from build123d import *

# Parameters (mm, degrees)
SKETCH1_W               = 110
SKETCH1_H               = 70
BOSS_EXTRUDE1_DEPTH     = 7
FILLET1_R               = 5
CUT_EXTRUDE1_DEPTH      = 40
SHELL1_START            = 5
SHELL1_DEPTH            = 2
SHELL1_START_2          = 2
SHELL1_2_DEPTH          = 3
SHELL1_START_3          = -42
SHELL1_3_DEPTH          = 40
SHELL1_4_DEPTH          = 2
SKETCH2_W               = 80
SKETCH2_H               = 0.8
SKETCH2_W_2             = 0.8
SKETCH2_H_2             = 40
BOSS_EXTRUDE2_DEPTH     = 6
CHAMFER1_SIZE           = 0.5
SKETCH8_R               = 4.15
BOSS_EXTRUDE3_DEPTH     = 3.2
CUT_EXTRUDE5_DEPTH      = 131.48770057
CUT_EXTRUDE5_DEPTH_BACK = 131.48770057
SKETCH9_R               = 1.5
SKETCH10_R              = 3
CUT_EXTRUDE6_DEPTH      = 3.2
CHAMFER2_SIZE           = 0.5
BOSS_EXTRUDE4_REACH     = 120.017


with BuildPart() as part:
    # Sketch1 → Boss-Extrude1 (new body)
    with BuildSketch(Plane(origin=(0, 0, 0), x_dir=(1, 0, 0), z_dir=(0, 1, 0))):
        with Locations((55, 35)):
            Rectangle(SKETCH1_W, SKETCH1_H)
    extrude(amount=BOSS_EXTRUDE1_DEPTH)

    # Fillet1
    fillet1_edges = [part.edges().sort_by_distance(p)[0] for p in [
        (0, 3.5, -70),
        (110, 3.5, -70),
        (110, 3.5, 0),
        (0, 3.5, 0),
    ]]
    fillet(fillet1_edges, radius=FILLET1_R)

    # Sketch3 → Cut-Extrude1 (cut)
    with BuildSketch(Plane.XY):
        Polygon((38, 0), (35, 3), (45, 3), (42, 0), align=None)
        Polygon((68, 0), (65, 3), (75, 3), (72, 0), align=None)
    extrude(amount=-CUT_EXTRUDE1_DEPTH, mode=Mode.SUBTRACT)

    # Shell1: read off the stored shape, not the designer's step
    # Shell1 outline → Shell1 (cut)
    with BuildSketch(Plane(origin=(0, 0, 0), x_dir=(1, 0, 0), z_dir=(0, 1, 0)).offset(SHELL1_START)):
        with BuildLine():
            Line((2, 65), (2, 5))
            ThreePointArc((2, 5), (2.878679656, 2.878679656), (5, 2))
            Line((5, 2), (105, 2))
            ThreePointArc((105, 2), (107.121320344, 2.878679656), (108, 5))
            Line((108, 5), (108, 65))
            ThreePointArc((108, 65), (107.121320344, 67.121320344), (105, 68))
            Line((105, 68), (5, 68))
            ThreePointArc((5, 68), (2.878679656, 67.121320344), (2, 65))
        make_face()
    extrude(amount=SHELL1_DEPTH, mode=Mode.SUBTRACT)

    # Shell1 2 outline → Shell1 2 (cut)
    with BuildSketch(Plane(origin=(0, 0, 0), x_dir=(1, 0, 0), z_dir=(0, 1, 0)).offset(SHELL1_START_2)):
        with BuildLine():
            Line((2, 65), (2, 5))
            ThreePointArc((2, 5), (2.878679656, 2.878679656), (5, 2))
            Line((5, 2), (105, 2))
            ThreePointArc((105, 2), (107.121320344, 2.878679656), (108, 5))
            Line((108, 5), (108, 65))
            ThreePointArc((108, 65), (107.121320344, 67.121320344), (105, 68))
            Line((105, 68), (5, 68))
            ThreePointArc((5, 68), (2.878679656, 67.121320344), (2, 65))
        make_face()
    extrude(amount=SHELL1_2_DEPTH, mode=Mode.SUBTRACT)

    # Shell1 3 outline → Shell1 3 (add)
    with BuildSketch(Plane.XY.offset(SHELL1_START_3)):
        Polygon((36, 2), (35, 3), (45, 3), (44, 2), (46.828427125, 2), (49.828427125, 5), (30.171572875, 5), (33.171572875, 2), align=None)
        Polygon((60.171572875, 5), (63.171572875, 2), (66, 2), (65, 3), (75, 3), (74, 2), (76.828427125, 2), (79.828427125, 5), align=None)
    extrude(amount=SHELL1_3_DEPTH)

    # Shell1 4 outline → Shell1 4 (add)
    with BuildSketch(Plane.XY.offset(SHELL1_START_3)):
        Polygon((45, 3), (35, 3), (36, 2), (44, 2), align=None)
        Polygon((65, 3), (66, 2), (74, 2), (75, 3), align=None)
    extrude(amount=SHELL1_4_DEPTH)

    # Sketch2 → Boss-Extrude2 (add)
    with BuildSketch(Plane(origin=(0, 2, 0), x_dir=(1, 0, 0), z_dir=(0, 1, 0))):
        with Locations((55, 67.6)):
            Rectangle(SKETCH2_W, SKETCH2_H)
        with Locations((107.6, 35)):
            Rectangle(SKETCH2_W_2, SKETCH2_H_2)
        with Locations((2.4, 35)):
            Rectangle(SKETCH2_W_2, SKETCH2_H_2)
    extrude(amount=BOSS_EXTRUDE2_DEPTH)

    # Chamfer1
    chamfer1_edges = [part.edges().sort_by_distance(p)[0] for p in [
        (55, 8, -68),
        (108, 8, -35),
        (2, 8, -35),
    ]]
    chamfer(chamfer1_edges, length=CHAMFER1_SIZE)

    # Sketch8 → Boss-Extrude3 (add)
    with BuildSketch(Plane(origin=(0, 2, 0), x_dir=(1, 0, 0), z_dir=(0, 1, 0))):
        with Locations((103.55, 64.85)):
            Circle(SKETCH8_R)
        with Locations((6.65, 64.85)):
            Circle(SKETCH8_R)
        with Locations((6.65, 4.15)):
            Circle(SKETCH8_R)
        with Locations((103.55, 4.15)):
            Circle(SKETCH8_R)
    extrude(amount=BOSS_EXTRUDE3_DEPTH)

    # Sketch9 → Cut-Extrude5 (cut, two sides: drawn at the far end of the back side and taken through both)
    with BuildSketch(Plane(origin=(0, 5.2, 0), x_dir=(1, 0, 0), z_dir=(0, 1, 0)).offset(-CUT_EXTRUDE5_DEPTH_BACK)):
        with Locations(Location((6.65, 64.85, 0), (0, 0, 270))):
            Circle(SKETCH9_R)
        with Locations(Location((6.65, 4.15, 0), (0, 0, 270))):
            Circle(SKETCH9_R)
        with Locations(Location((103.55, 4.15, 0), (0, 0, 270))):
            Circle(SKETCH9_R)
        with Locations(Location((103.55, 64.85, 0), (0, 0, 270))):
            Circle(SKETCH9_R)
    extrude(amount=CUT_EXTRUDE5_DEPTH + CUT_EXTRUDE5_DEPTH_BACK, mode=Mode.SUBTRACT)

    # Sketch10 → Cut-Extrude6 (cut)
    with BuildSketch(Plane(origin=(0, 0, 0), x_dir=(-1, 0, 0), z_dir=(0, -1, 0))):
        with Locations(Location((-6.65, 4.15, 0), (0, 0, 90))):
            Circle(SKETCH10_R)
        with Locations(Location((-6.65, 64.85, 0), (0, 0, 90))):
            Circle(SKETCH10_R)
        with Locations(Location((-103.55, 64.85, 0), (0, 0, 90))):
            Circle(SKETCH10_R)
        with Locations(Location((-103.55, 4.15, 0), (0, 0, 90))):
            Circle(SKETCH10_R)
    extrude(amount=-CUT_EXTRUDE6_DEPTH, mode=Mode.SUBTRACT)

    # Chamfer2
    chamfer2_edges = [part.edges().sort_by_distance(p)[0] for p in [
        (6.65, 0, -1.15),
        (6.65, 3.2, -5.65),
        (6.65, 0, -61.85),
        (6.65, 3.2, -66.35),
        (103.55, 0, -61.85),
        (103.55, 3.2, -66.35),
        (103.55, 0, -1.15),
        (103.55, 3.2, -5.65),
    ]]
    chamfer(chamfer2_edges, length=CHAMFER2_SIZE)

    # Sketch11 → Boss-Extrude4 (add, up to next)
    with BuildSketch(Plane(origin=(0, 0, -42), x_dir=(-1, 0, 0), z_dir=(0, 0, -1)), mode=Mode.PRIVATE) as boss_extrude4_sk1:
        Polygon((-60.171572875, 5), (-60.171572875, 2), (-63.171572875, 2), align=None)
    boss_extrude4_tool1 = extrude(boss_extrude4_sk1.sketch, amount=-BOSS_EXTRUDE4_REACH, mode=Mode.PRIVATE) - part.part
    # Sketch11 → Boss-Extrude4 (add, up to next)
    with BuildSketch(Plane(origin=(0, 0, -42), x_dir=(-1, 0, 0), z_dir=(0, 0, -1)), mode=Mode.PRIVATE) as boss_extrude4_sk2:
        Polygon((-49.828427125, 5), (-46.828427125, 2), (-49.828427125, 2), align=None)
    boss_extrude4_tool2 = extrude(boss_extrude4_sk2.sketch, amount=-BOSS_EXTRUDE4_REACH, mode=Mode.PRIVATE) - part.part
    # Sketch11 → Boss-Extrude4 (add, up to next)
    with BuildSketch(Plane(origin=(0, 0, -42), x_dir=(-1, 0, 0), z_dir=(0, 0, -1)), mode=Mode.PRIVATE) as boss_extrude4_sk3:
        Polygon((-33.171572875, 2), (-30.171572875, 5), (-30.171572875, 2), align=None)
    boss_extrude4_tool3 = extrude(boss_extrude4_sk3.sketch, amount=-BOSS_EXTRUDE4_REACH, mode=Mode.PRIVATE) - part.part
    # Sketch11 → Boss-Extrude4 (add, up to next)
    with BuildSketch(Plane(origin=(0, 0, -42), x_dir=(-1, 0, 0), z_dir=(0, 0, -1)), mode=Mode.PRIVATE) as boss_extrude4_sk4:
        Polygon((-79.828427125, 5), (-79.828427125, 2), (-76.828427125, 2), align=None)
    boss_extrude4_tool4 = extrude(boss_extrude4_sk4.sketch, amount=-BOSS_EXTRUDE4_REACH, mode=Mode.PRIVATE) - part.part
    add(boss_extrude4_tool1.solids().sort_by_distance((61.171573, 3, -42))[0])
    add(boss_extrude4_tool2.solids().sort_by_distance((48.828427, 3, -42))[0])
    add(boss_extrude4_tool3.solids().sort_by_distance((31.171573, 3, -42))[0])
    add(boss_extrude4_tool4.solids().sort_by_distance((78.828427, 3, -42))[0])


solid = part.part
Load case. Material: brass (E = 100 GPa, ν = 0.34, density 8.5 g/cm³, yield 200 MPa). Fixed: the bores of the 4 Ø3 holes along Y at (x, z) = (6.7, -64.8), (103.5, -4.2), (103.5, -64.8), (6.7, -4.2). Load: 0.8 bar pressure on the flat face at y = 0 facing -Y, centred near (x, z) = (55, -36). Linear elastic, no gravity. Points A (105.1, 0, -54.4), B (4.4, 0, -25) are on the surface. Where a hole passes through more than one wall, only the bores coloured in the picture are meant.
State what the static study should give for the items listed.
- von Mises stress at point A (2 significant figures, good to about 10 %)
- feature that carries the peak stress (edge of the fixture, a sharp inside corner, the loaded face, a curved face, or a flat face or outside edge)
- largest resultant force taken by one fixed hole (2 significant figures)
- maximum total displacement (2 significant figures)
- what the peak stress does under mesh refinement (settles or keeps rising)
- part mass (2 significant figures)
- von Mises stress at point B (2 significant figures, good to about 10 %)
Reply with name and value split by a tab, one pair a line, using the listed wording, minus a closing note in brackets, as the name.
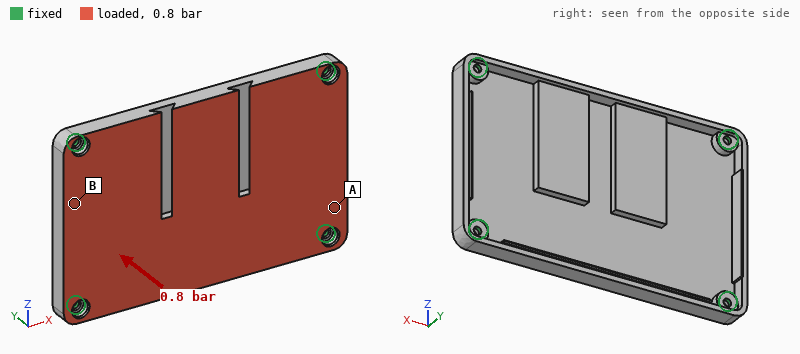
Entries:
von Mises stress at point A	18 MPa
feature that carries the peak stress	edge of the fixture
largest resultant force taken by one fixed hole	320 N
maximum total displacement	0.13 mm
what the peak stress does under mesh refinement	keeps rising
part mass	190 g
von Mises stress at point B	8.6 MPa
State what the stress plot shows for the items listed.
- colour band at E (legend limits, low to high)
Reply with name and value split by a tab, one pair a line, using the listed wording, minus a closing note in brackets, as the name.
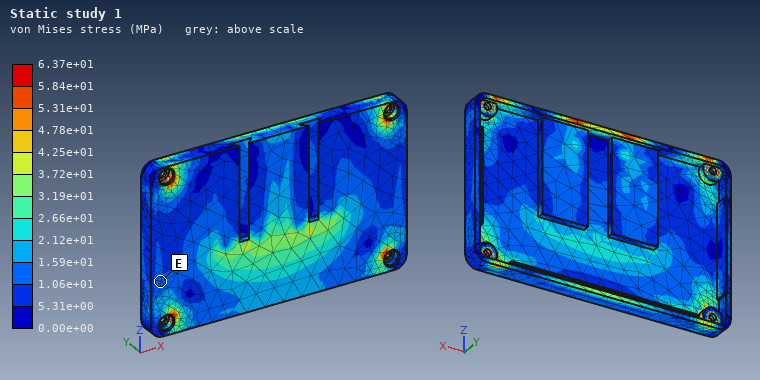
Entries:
colour band at E	1.06e+01 to 1.59e+01 MPa
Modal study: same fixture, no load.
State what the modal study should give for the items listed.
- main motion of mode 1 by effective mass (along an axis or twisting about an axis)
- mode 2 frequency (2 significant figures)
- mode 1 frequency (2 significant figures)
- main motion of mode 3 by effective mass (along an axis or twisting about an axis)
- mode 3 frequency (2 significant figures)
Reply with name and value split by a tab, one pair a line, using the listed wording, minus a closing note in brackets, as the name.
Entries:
main motion of mode 1 by effective mass	along Y
mode 2 frequency	1600 Hz
mode 1 frequency	890 Hz
main motion of mode 3 by effective mass	twisting about Z
mode 3 frequency	2100 Hz
